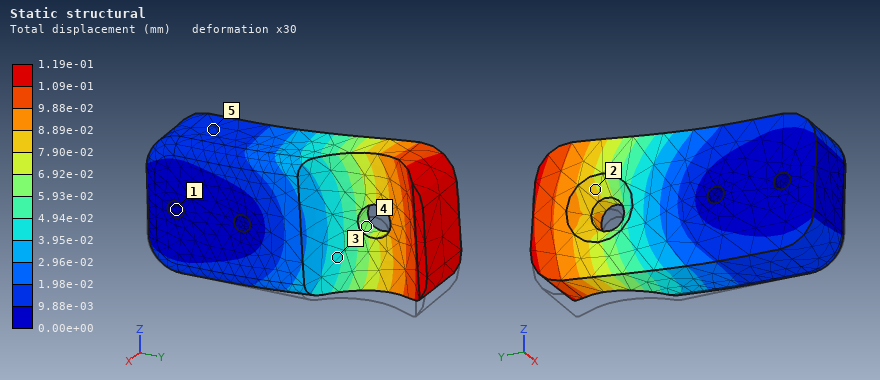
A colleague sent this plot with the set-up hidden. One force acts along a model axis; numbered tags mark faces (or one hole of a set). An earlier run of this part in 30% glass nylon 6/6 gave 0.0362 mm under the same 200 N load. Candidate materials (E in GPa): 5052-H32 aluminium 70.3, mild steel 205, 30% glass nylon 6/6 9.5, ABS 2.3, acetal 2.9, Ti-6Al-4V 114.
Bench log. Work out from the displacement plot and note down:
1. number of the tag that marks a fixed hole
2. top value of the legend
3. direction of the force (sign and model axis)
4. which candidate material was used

1
1.19e-01 mm
+Z
acetal
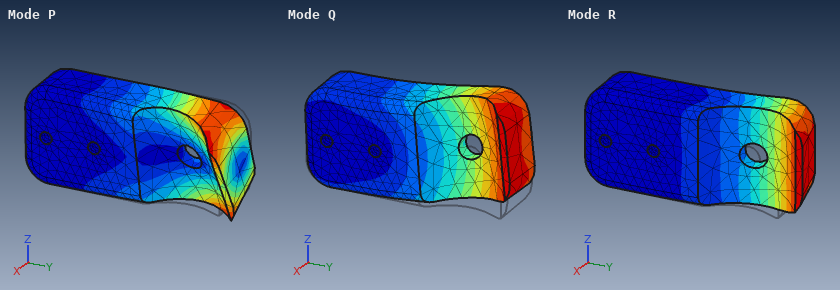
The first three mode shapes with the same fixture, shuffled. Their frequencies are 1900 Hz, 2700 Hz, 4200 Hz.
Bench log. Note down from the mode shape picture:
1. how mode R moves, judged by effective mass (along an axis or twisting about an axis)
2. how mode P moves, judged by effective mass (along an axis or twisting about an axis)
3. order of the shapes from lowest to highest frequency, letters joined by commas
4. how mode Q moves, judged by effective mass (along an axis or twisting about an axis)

along X
twisting about Y
R, Q, P
along Z
